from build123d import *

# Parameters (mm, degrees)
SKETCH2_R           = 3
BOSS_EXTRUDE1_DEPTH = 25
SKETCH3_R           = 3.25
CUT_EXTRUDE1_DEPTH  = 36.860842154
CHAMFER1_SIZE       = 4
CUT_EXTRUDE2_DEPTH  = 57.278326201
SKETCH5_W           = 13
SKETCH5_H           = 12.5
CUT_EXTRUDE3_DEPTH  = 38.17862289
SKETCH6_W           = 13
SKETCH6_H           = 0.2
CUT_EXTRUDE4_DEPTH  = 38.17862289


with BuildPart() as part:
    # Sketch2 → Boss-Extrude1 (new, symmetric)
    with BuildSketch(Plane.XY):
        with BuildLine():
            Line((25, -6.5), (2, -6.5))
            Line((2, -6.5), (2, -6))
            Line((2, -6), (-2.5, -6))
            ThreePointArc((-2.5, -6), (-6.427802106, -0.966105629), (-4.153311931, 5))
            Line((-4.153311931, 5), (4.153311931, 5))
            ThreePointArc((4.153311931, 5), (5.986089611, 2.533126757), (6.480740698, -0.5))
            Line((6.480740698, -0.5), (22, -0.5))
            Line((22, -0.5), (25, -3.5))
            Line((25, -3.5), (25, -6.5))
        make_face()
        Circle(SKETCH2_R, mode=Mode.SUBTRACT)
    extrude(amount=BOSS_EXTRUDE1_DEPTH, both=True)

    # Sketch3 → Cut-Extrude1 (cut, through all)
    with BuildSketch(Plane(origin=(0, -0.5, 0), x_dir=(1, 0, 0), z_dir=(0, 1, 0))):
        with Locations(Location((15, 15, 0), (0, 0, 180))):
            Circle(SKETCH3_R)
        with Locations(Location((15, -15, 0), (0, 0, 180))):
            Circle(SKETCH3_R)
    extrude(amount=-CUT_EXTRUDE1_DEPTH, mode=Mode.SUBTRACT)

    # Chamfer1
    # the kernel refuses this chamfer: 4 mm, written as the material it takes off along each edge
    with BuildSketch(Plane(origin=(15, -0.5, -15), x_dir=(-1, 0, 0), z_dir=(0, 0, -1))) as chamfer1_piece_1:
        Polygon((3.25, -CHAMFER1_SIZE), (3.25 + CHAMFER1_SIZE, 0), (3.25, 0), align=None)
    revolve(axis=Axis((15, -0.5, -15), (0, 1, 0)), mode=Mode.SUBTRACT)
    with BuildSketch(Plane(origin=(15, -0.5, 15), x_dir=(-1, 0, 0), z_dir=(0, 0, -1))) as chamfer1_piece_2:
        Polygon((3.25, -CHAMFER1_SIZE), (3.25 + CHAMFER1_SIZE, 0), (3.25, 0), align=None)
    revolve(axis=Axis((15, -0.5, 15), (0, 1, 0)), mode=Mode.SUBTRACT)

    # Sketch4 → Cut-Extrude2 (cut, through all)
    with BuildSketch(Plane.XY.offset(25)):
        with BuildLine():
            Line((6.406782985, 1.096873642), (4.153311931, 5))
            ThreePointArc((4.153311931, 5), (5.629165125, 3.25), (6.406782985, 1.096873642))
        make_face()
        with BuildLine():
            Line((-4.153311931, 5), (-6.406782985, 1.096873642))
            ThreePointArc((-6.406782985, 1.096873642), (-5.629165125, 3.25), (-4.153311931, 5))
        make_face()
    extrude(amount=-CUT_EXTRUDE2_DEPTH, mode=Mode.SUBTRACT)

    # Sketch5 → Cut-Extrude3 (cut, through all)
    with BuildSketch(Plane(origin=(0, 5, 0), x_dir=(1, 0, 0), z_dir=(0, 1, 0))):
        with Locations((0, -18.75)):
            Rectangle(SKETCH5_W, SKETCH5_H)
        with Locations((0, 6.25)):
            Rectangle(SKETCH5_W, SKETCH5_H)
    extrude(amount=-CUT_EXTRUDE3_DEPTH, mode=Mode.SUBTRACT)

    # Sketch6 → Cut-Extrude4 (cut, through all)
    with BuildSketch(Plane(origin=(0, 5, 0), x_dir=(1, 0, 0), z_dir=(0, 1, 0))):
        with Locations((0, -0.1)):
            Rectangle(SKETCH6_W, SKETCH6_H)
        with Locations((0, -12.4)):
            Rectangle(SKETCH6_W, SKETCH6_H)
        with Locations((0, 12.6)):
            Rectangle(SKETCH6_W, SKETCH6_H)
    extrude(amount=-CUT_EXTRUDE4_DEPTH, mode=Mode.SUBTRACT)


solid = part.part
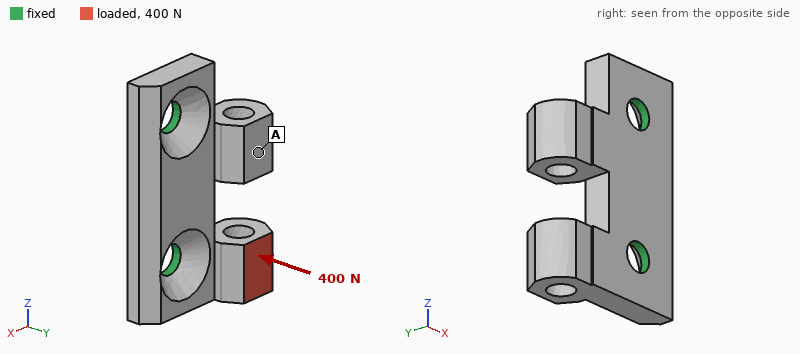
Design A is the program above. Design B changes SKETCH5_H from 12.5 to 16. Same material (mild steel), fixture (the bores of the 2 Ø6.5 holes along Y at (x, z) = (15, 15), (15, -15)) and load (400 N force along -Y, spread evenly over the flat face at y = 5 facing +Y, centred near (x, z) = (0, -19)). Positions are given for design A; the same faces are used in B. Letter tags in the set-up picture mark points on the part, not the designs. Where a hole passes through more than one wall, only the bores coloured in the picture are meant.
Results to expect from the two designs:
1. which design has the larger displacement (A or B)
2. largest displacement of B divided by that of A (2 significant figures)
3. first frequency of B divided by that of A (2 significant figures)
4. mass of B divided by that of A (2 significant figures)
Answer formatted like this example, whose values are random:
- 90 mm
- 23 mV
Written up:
- B
- 1.1
- 1.0
- 0.93
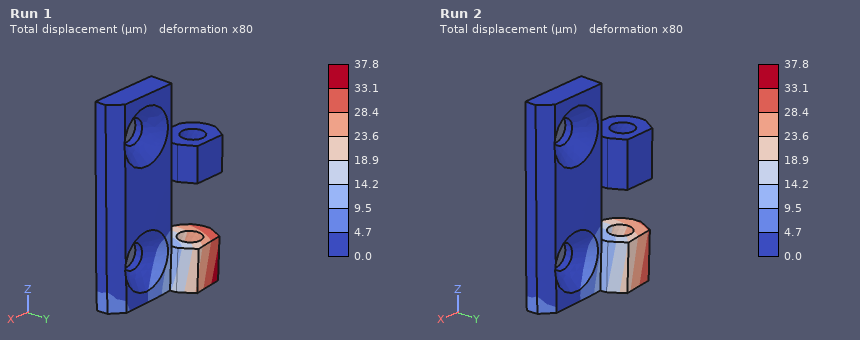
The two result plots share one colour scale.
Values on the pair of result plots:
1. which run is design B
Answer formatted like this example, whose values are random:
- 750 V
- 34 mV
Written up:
- Run 1
